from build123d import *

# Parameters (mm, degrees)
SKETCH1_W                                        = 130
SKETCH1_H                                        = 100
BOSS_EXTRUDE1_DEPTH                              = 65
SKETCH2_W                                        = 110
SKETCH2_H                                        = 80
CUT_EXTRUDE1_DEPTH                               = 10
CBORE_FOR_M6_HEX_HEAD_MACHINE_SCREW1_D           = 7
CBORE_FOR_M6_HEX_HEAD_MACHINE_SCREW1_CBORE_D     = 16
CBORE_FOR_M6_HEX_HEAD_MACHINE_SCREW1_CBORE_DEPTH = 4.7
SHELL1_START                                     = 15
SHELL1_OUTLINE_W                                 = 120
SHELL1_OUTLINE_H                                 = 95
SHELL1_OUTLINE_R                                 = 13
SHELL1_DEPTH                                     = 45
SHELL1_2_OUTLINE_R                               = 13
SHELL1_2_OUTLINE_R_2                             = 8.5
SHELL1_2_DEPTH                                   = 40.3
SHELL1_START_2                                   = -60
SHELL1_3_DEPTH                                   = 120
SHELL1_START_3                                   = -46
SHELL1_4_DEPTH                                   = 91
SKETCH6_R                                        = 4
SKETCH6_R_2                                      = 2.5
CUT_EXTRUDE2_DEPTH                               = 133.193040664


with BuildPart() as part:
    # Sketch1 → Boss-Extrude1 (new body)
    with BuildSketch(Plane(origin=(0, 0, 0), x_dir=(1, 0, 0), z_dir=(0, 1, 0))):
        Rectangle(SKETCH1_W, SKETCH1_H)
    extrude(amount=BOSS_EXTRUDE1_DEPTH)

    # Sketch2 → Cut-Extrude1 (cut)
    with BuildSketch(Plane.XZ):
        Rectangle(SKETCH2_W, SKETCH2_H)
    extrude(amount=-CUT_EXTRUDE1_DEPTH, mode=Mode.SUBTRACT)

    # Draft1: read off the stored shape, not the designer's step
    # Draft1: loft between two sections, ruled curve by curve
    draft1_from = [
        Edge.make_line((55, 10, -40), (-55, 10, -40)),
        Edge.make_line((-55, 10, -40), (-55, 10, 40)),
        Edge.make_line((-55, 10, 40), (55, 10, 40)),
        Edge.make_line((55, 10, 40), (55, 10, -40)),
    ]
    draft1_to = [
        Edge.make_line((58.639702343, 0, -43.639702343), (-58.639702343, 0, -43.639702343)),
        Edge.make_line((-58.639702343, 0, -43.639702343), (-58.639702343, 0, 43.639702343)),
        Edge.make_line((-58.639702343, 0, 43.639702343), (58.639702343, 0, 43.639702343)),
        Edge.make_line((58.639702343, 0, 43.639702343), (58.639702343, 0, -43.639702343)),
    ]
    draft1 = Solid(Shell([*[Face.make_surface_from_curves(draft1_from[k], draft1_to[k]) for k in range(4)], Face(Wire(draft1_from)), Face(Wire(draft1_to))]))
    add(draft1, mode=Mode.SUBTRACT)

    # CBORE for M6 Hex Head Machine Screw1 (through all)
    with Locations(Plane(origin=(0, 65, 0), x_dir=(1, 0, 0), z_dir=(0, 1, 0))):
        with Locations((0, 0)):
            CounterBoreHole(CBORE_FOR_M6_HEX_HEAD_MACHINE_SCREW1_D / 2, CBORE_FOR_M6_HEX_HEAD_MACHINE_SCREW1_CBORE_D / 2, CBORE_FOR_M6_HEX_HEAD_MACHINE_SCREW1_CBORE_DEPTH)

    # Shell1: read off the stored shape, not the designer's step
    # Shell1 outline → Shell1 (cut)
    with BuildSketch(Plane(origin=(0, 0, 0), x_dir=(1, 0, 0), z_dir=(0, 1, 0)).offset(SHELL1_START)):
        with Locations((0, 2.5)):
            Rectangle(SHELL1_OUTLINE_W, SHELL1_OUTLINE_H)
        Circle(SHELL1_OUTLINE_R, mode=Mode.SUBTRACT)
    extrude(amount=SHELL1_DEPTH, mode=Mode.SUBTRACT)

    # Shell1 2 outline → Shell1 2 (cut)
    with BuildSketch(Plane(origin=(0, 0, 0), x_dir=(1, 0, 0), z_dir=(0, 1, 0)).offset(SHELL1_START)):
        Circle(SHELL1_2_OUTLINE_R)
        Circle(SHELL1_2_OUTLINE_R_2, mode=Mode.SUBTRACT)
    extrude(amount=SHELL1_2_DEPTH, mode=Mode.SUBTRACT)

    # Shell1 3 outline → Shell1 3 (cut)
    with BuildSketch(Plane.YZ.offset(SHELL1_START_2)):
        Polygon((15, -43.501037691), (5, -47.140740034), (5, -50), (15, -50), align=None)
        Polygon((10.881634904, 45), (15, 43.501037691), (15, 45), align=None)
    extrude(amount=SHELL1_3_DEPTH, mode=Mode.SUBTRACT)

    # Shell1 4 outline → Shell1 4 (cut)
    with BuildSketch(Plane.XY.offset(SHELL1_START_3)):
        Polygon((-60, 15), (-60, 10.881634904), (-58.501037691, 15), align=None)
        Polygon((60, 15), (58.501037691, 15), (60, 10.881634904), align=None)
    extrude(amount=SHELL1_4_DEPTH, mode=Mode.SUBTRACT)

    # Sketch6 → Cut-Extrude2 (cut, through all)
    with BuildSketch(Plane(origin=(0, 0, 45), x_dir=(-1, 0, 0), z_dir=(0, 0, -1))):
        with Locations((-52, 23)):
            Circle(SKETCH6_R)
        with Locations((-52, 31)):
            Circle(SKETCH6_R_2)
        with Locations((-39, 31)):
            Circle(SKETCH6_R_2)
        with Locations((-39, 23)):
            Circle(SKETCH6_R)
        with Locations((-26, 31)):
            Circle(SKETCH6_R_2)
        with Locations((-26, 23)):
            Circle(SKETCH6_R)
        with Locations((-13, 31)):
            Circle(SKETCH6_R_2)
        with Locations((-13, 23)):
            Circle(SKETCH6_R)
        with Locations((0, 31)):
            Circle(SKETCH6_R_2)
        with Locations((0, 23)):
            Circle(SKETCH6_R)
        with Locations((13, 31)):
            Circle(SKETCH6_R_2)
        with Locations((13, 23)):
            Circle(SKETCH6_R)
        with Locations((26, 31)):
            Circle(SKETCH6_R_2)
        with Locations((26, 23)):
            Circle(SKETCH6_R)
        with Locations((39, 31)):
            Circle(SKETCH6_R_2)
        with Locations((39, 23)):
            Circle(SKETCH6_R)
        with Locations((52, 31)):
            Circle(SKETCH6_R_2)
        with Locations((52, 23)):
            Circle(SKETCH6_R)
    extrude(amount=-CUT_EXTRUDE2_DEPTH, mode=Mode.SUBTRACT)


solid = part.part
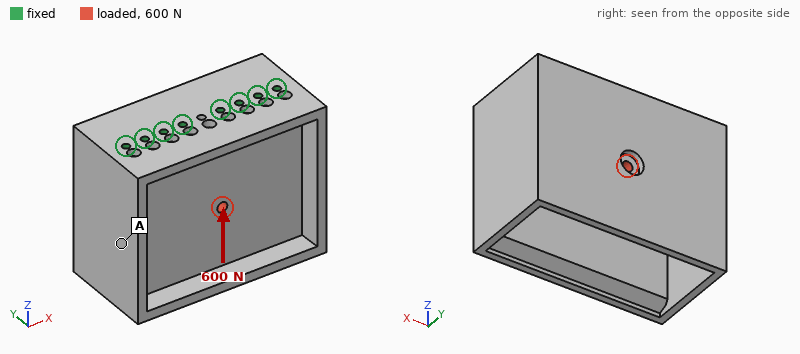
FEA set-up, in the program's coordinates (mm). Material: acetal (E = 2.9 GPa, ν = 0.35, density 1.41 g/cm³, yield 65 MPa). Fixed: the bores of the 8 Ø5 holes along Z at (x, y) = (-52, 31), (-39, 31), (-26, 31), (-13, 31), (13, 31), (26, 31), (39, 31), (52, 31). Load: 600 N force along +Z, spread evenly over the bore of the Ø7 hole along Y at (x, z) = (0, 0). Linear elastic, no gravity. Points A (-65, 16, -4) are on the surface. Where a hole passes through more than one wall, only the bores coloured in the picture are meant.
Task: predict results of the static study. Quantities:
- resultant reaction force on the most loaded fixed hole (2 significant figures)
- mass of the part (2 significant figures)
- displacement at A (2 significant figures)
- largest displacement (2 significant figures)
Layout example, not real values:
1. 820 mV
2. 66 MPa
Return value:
1. 220 N
2. 330 g
3. 0.15 mm
4. 0.33 mm
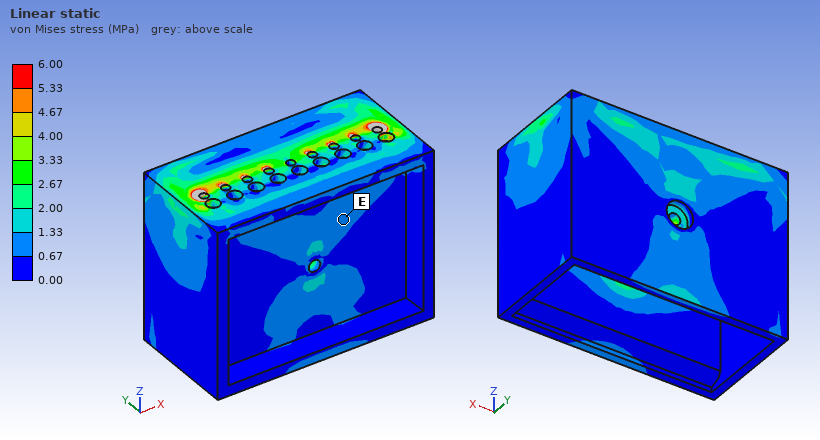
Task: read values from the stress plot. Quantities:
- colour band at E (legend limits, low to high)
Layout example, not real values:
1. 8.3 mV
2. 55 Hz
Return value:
1. 0.67 to 1.33 MPa
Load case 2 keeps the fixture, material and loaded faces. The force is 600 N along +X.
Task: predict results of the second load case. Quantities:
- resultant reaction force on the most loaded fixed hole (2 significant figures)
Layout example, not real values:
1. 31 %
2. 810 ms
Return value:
1. 250 N
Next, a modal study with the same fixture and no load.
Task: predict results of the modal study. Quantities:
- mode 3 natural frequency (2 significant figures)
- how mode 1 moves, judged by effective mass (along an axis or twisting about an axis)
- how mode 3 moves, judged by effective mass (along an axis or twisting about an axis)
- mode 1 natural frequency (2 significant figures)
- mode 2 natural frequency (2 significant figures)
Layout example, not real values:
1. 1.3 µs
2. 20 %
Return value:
1. 540 Hz
2. along Y
3. along X
4. 140 Hz
5. 410 Hz
